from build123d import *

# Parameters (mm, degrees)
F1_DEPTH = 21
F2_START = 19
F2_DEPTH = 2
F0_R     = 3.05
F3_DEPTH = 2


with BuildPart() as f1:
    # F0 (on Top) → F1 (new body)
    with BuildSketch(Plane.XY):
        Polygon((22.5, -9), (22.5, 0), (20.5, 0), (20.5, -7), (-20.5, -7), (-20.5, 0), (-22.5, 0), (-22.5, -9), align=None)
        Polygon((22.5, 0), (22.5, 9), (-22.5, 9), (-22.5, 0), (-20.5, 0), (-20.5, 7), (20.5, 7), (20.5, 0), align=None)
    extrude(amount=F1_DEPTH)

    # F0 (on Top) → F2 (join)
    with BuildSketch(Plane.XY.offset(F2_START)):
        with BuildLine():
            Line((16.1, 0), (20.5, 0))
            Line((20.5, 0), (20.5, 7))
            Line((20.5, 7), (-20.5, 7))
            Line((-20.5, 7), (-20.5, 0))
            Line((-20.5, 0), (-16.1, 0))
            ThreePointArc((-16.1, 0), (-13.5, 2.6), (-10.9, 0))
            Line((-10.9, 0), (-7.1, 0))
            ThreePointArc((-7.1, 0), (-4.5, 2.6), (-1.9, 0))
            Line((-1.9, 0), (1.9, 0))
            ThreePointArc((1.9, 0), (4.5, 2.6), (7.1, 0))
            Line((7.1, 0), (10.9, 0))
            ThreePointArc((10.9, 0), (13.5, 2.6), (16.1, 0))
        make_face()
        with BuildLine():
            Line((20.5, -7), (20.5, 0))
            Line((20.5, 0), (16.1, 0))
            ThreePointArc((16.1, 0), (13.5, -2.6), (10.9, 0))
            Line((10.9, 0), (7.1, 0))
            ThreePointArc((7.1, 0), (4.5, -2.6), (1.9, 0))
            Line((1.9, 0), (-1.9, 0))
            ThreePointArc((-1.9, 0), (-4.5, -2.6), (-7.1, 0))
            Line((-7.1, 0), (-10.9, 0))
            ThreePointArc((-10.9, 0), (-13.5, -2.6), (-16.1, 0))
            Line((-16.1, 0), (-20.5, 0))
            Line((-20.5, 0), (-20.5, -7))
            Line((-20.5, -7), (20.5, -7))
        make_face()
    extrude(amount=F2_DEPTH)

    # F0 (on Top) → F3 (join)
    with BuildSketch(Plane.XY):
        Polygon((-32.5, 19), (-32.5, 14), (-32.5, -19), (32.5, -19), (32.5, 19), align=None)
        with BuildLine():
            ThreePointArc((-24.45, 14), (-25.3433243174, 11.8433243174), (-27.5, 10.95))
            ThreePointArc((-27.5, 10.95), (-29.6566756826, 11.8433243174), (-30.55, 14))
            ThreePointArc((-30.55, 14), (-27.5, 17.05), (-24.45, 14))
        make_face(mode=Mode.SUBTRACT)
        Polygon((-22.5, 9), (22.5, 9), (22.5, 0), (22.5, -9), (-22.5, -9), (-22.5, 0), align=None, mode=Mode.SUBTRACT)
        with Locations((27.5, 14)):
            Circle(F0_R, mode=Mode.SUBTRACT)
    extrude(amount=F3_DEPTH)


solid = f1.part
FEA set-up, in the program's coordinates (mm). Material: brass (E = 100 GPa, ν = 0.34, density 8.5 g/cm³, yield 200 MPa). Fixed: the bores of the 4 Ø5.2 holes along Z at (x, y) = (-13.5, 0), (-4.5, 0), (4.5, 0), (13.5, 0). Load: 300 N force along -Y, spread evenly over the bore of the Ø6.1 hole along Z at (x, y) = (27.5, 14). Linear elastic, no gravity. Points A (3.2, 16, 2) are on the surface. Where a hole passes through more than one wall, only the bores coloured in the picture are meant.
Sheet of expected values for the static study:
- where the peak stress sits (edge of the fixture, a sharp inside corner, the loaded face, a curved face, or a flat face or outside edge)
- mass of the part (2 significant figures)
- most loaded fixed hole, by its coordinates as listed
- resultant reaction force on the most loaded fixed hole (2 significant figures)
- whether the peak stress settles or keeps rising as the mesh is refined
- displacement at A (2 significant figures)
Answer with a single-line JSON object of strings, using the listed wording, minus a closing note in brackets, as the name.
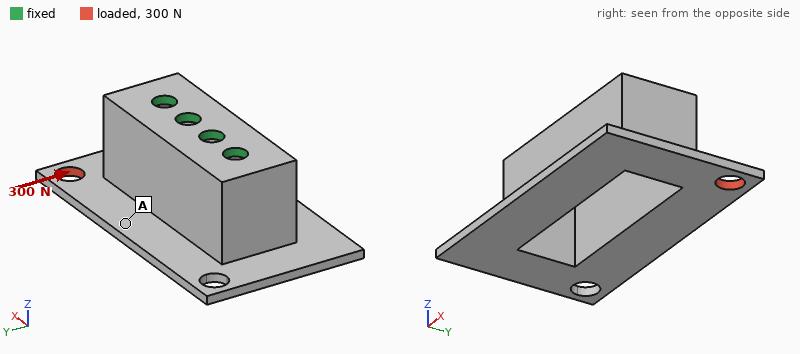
{"where the peak stress sits": "edge of the fixture", "mass of the part": "78 g", "most loaded fixed hole, by its coordinates as listed": "(13.5, 0)", "resultant reaction force on the most loaded fixed hole": "460 N", "whether the peak stress settles or keeps rising as the mesh is refined": "keeps rising", "displacement at A": "38 µm"}
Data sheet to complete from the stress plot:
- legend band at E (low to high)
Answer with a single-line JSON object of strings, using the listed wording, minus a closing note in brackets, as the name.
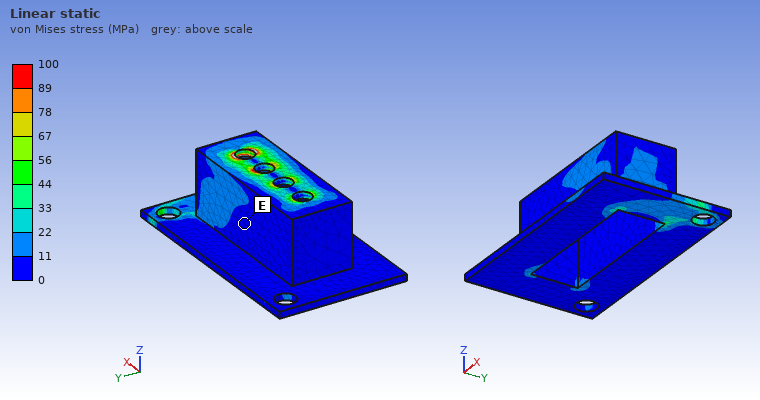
{"legend band at E": "0 to 11 MPa"}
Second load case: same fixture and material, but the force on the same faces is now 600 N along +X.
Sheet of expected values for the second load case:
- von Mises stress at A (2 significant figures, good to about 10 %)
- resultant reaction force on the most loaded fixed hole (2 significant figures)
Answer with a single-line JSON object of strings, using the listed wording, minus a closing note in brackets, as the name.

{"von Mises stress at A": "16 MPa", "resultant reaction force on the most loaded fixed hole": "430 N"}
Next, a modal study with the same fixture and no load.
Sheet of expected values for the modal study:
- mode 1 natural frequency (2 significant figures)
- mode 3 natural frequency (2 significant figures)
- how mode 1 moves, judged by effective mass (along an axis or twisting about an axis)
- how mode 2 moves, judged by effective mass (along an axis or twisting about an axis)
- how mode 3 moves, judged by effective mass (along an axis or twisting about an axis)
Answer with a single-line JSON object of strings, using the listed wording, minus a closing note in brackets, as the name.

{"mode 1 natural frequency": "2100 Hz", "mode 3 natural frequency": "4200 Hz", "how mode 1 moves, judged by effective mass": "along Y", "how mode 2 moves, judged by effective mass": "along X", "how mode 3 moves, judged by effective mass": "twisting about Z"}
